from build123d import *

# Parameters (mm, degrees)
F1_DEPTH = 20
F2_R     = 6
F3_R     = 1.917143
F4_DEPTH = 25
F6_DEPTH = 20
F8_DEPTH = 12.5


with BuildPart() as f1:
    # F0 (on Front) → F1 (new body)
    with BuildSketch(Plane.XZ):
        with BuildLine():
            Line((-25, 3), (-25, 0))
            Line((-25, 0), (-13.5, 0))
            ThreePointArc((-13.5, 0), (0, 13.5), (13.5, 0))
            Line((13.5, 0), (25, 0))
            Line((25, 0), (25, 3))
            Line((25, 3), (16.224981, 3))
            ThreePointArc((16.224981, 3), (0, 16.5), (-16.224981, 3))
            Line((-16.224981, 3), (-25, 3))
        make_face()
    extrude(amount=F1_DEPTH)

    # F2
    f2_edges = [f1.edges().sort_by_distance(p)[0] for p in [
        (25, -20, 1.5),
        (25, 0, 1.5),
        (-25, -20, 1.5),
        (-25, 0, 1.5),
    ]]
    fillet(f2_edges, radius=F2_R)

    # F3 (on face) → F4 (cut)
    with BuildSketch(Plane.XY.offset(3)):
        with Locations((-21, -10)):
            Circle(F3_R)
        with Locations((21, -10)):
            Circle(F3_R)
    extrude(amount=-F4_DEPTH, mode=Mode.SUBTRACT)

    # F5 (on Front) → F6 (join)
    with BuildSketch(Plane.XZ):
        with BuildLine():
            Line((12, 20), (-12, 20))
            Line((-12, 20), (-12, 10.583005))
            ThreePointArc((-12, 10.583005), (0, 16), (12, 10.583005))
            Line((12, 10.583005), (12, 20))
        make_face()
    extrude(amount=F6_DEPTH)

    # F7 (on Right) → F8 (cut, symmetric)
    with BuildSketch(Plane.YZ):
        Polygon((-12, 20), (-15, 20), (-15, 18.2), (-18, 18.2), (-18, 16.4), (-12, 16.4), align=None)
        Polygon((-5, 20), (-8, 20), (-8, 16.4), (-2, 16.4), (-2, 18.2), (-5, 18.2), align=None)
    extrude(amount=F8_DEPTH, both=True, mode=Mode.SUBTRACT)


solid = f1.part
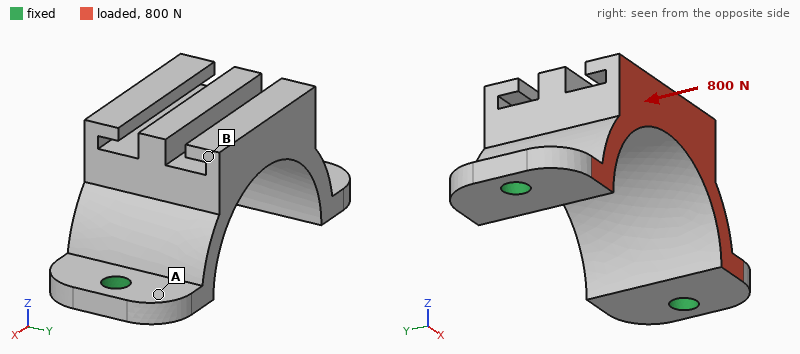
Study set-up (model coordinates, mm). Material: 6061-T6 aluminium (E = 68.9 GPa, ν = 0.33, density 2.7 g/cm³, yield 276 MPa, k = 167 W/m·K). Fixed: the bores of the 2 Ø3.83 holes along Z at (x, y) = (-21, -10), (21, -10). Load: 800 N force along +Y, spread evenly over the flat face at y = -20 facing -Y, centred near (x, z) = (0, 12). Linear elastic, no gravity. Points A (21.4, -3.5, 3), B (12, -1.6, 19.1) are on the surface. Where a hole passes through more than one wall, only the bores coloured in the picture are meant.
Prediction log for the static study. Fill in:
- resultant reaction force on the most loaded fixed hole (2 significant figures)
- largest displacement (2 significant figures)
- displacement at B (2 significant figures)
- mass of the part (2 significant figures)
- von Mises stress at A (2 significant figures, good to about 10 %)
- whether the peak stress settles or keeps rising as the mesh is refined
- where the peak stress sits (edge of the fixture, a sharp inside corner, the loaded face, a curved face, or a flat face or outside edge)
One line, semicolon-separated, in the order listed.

400 N; 0.13 mm; 0.11 mm; 14 g; 41 MPa; keeps rising; edge of the fixture
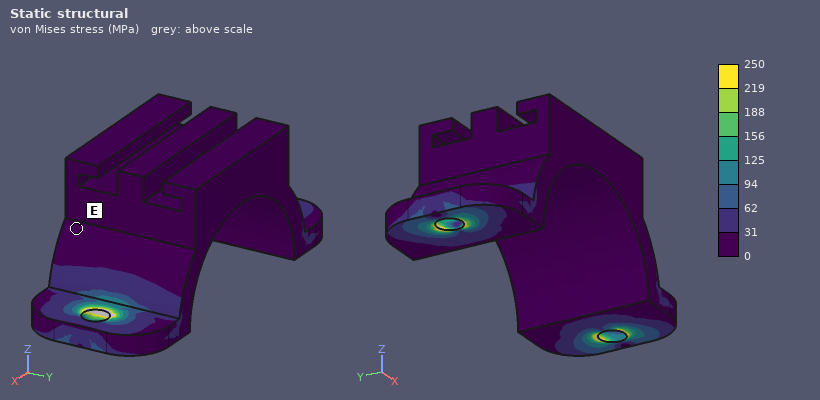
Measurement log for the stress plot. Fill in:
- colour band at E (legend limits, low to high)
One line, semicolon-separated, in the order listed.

0 to 31 MPa
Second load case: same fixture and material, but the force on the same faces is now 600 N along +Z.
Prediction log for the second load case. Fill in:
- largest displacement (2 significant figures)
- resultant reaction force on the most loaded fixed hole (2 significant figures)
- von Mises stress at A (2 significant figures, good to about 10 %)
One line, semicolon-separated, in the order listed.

81 µm; 350 N; 24 MPa
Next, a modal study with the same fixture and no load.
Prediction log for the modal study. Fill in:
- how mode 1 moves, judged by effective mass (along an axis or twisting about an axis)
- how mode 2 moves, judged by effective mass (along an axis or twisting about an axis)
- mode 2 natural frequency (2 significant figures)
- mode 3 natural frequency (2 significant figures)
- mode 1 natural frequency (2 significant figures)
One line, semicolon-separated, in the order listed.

along Y; along X; 12 kHz; 13 kHz; 4200 Hz
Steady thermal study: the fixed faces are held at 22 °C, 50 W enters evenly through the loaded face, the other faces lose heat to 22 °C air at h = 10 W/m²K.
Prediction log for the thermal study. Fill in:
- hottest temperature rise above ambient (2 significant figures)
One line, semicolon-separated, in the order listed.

58 K
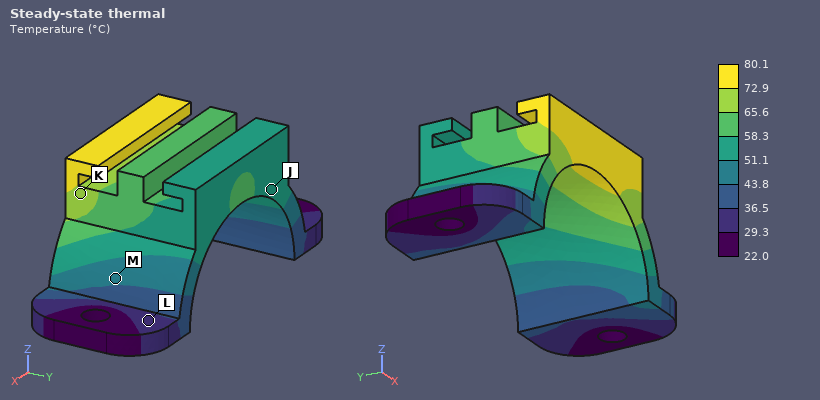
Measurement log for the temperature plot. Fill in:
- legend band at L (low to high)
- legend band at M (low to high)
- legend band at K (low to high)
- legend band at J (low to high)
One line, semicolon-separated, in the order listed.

29.3 to 36.5 °C; 43.8 to 51.1 °C; 65.6 to 72.9 °C; 51.1 to 58.3 °C
